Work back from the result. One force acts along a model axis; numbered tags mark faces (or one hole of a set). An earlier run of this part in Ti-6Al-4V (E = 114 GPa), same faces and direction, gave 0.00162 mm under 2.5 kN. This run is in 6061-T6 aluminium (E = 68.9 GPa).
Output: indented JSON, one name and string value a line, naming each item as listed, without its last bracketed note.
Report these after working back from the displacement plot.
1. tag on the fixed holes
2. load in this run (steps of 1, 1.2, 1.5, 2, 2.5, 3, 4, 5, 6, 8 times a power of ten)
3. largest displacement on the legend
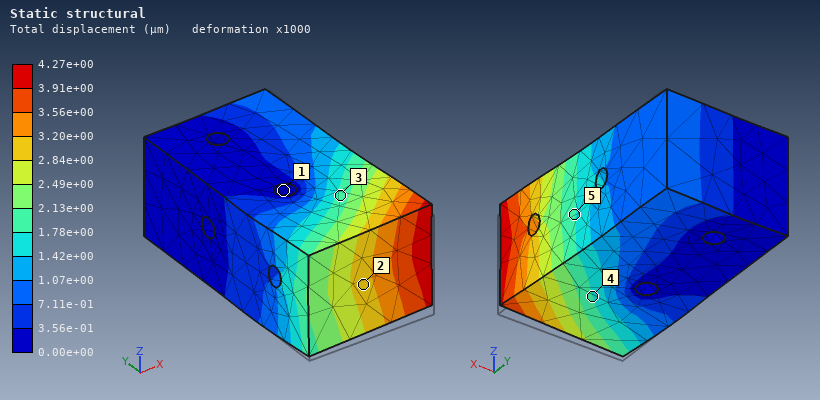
{
  "tag on the fixed holes": "1",
  "load in this run": "4 kN",
  "largest displacement on the legend": "4.27e+00 µm"
}
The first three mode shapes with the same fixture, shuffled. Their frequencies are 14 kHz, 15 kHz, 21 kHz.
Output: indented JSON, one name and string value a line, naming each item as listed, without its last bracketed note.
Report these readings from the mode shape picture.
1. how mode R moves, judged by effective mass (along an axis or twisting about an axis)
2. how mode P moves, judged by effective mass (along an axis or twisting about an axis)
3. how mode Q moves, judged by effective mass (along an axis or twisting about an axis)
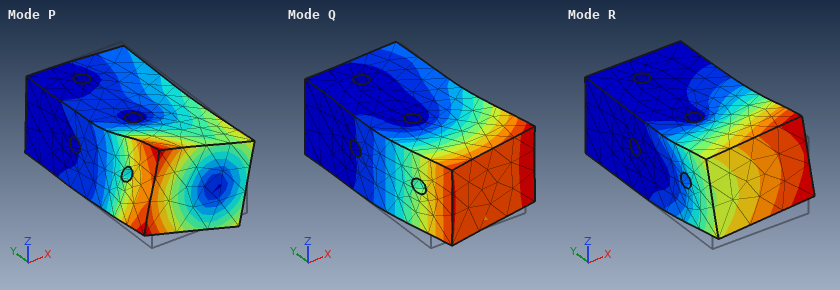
{
  "how mode R moves, judged by effective mass": "along Z",
  "how mode P moves, judged by effective mass": "twisting about Y",
  "how mode Q moves, judged by effective mass": "along X"
}
